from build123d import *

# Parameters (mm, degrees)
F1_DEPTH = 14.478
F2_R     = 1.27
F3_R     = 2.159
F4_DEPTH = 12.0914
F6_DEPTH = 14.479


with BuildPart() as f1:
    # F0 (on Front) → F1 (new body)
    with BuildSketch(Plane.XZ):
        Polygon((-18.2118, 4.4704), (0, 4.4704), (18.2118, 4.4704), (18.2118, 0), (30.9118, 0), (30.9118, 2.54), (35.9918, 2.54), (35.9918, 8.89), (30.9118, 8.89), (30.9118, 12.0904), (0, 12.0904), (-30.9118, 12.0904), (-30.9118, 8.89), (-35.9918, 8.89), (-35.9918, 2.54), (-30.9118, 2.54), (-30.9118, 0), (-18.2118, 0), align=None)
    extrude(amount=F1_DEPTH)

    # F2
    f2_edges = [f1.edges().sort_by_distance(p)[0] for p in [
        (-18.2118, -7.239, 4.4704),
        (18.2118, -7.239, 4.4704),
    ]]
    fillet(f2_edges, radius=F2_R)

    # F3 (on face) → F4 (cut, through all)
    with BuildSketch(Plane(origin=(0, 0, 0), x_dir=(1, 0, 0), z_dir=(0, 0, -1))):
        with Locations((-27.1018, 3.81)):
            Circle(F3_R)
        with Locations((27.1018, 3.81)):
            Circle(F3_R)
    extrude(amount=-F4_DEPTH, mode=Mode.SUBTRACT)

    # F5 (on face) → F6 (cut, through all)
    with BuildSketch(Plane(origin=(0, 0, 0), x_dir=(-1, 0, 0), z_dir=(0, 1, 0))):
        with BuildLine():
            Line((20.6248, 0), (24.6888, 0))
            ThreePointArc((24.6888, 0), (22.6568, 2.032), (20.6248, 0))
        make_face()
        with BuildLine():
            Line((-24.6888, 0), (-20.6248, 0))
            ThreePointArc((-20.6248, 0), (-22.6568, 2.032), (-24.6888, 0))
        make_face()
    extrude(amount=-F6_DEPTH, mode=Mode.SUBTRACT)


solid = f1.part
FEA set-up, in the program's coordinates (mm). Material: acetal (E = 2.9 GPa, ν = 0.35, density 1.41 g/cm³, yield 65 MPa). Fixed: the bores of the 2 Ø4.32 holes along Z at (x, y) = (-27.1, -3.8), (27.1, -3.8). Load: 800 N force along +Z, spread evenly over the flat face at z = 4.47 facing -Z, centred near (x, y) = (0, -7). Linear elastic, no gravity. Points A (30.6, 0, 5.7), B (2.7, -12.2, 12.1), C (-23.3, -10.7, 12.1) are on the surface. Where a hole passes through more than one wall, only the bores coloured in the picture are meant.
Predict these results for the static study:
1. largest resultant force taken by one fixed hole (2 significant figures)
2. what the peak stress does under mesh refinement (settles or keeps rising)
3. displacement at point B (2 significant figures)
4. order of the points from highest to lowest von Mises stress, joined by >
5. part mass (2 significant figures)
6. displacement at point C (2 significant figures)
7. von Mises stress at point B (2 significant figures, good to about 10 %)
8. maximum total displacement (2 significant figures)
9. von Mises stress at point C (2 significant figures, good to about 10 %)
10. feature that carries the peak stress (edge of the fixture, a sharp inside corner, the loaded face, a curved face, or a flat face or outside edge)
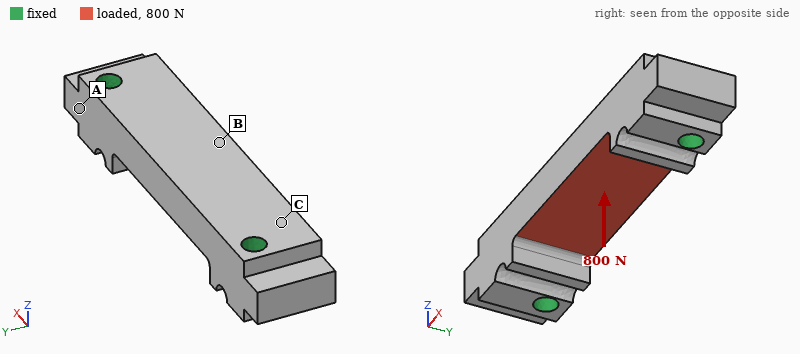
420 N
keeps rising
0.26 mm
B > C > A
13 g
0.044 mm
15 MPa
0.28 mm
8.6 MPa
edge of the fixture
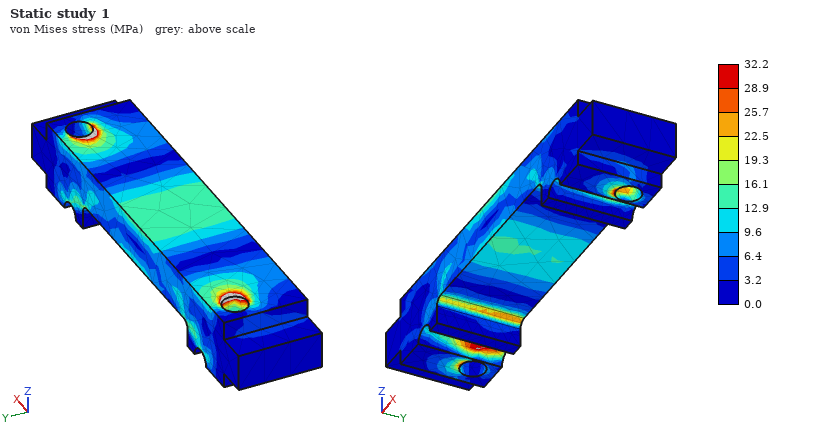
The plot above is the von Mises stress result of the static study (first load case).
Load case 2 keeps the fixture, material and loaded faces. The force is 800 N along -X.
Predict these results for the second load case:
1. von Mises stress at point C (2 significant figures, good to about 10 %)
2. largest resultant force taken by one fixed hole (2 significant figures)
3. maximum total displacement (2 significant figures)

2.1 MPa
410 N
37 µm
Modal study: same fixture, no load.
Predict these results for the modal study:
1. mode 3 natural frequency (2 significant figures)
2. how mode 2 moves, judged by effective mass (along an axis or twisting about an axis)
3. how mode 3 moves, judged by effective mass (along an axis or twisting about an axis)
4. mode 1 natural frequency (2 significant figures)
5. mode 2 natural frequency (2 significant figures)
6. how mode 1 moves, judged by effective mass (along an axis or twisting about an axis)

7400 Hz
along Y
twisting about X
4100 Hz
4600 Hz
along Z
